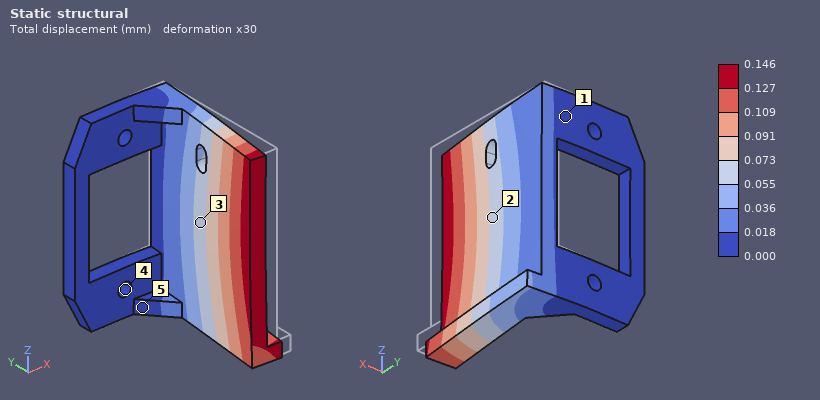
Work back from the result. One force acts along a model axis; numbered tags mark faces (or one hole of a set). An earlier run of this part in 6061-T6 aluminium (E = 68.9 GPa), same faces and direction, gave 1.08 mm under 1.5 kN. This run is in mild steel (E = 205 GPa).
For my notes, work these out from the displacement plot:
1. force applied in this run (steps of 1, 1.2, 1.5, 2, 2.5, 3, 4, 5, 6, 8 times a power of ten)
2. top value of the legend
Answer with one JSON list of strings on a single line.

["600 N", "0.146 mm"]
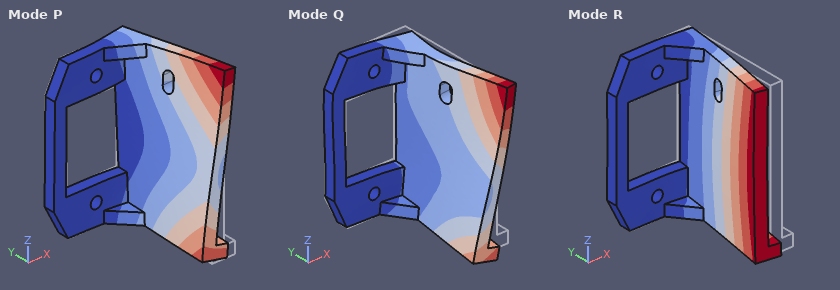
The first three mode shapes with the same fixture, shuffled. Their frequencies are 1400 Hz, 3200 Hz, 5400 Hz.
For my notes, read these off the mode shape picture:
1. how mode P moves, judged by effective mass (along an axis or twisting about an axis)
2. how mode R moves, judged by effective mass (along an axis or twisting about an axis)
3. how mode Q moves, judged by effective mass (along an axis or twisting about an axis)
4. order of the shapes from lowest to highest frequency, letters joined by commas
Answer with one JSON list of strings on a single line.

["along Z", "along X", "along Z", "R, P, Q"]
